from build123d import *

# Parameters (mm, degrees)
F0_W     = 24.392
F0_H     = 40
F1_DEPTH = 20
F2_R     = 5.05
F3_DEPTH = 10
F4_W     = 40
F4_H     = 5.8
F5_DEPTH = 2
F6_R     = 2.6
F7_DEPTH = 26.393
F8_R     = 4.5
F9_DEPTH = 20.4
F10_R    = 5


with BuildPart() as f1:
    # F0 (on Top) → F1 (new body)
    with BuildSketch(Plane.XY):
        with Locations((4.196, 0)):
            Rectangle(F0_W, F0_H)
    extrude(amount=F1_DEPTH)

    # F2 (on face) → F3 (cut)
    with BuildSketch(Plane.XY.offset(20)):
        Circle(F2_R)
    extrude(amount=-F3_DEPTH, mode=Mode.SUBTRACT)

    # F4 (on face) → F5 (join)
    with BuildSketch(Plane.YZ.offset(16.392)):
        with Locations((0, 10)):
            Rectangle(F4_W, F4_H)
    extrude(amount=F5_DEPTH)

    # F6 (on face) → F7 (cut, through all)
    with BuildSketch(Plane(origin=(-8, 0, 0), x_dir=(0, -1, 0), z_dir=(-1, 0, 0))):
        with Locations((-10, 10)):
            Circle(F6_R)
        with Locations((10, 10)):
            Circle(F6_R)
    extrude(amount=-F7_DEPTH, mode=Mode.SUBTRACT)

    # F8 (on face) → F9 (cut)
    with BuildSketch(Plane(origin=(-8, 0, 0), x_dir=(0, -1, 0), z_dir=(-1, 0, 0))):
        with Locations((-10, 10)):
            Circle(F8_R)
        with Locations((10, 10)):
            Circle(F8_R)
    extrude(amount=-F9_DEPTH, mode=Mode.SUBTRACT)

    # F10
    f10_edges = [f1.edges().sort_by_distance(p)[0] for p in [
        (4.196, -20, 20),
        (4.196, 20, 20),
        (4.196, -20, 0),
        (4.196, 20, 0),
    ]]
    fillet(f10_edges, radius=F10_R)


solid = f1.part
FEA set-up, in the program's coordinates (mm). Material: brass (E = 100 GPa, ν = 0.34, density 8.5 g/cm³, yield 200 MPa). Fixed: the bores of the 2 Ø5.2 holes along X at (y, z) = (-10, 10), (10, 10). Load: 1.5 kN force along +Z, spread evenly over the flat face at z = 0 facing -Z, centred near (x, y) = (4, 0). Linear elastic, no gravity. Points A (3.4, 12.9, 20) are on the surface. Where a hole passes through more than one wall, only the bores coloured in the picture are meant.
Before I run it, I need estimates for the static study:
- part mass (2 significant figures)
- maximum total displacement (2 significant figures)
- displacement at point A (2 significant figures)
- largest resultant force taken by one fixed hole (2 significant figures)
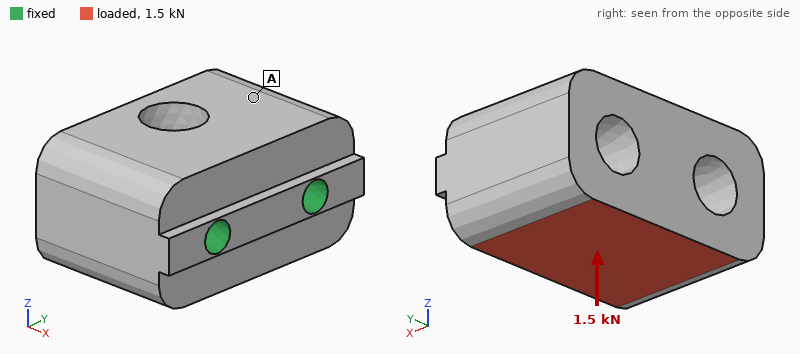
130 g
20 µm
12 µm
750 N
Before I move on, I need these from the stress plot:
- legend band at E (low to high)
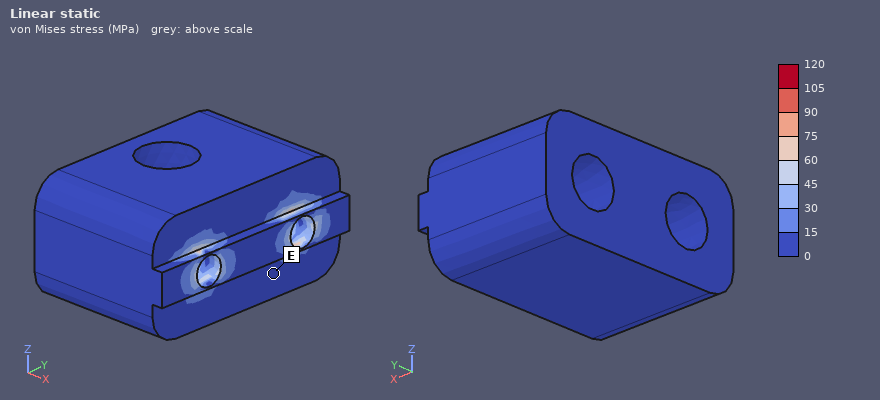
0 to 15 MPa
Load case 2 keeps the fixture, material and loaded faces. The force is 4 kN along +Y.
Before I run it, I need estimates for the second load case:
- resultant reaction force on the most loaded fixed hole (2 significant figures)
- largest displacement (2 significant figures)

3.1 kN
14 µm
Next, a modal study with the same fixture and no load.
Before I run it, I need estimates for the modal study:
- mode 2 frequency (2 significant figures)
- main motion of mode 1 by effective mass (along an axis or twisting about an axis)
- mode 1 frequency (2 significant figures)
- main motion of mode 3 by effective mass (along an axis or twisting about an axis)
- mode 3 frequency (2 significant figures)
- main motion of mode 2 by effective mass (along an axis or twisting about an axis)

9700 Hz
along Z
4600 Hz
twisting about X
12 kHz
along Y
